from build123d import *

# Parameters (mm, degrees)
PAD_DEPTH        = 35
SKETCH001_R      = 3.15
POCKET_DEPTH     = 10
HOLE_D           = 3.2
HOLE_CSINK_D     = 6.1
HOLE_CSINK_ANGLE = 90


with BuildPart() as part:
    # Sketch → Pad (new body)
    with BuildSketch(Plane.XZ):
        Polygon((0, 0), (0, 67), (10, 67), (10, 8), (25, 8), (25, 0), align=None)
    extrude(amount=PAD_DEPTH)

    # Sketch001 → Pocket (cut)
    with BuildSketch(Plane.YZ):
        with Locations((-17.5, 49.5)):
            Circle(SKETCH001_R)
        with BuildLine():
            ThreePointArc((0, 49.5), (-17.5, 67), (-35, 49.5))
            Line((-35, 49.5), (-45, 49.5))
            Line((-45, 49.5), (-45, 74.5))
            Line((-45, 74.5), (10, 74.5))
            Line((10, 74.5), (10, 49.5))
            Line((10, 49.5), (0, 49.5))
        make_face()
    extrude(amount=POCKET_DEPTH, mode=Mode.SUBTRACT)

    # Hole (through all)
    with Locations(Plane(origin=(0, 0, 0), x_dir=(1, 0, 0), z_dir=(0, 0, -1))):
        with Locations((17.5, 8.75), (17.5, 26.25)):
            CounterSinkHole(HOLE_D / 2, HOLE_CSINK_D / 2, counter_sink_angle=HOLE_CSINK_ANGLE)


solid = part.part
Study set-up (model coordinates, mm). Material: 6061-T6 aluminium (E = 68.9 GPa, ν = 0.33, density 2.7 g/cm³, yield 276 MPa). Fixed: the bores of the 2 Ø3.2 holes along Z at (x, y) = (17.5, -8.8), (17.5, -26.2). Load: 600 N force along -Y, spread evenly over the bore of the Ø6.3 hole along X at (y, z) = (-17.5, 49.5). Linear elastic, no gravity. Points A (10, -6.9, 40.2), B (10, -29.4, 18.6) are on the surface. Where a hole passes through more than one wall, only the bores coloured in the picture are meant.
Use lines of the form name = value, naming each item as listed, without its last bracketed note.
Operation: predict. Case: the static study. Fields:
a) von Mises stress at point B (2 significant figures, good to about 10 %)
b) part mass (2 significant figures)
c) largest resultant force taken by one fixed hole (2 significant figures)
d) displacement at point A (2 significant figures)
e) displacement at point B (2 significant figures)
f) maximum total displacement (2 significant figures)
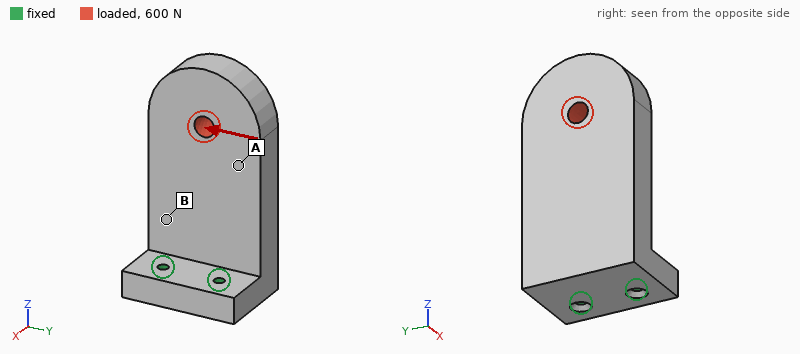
von Mises stress at point B = 13 MPa
part mass = 70 g
largest resultant force taken by one fixed hole = 1.3 kN
displacement at point A = 48 µm
displacement at point B = 23 µm
maximum total displacement = 80 µm
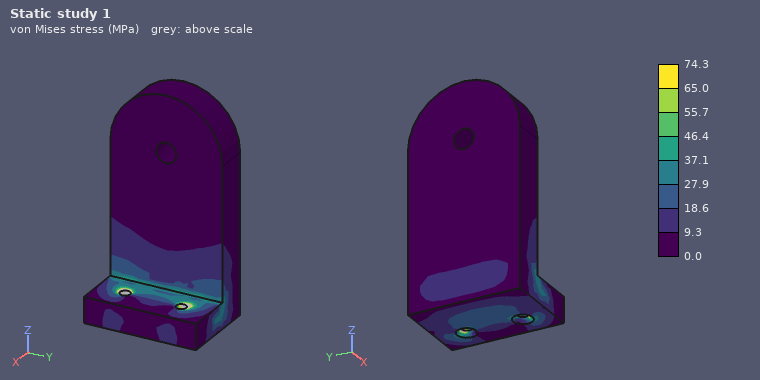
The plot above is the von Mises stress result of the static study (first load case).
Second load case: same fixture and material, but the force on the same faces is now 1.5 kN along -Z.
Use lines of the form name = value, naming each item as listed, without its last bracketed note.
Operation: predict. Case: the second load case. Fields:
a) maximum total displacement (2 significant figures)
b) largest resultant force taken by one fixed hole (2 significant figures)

maximum total displacement = 0.12 mm
largest resultant force taken by one fixed hole = 750 N
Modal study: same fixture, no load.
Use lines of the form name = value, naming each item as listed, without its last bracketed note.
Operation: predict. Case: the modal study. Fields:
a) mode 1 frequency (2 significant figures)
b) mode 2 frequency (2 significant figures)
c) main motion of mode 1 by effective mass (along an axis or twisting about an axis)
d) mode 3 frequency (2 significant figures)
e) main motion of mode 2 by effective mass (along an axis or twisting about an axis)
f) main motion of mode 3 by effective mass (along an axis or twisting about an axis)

mode 1 frequency = 1400 Hz
mode 2 frequency = 2800 Hz
main motion of mode 1 by effective mass = along X
mode 3 frequency = 7200 Hz
main motion of mode 2 by effective mass = along Y
main motion of mode 3 by effective mass = twisting about Z
